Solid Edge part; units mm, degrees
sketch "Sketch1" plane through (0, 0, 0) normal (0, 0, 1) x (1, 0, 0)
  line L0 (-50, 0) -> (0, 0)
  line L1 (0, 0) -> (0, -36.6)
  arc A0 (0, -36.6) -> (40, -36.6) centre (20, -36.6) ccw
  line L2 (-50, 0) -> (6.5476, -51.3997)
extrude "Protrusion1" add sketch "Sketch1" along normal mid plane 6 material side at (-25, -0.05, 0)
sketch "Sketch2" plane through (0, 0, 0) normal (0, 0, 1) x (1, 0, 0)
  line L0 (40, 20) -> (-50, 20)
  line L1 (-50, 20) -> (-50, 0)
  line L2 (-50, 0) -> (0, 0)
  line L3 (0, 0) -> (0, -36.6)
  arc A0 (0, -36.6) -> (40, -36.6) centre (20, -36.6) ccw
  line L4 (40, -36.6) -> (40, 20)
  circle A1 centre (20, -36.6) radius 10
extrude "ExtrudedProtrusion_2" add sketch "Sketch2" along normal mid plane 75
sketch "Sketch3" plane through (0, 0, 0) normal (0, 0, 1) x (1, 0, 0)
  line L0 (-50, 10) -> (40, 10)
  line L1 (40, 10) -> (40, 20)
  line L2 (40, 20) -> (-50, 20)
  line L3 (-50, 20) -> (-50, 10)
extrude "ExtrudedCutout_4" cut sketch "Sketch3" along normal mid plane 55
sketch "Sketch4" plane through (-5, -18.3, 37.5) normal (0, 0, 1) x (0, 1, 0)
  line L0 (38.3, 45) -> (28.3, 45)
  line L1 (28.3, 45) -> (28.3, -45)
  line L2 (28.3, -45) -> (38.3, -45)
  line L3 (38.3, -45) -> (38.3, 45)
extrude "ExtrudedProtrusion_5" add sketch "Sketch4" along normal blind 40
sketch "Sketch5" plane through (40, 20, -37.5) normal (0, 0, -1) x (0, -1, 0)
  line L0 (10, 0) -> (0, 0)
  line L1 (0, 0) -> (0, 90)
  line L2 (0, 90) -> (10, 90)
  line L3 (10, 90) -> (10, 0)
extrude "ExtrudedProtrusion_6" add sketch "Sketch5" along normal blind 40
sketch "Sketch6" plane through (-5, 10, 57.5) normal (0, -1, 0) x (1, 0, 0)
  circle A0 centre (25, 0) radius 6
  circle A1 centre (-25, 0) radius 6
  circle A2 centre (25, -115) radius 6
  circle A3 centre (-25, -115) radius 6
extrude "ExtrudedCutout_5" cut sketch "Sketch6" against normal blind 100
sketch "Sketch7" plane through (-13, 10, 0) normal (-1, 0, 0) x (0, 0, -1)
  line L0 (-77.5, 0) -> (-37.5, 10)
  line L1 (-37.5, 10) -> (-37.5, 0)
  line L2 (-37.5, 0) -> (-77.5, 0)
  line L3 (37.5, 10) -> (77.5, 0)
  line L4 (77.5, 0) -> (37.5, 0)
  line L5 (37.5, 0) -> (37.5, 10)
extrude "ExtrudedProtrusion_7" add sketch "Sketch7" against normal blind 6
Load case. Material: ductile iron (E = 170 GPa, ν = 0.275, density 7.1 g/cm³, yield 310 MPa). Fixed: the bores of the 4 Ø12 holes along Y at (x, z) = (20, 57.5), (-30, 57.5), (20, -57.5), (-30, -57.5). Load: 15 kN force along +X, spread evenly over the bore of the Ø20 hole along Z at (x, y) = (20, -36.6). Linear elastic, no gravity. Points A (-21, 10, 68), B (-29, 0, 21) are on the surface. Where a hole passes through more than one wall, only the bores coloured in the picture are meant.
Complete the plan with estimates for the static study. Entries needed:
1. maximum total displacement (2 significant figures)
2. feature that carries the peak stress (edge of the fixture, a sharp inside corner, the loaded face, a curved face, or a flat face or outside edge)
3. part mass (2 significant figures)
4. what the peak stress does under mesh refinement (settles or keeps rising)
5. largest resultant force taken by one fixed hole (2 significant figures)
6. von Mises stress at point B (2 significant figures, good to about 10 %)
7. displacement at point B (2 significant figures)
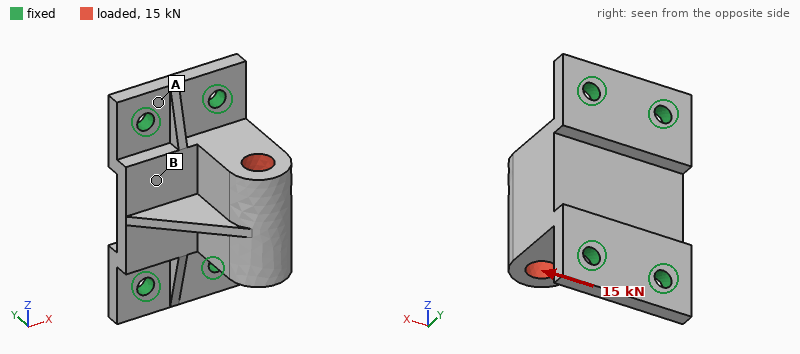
0.11 mm
edge of the fixture
2.1 kg
keeps rising
13 kN
38 MPa
0.032 mm
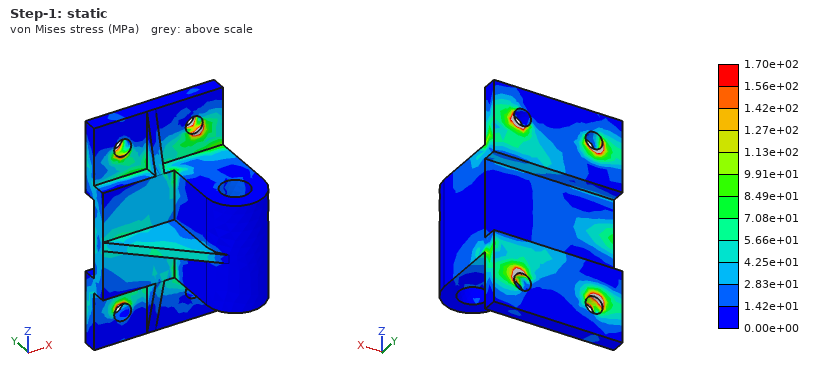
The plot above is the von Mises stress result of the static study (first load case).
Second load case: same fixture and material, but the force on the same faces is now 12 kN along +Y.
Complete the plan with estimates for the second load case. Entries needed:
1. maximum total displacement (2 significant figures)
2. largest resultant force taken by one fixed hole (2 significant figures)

31 µm
7.2 kN
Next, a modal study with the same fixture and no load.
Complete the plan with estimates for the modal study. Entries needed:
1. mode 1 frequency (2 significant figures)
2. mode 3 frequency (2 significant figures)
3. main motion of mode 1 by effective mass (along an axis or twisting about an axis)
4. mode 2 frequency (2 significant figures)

2300 Hz
4100 Hz
along X
4000 Hz
